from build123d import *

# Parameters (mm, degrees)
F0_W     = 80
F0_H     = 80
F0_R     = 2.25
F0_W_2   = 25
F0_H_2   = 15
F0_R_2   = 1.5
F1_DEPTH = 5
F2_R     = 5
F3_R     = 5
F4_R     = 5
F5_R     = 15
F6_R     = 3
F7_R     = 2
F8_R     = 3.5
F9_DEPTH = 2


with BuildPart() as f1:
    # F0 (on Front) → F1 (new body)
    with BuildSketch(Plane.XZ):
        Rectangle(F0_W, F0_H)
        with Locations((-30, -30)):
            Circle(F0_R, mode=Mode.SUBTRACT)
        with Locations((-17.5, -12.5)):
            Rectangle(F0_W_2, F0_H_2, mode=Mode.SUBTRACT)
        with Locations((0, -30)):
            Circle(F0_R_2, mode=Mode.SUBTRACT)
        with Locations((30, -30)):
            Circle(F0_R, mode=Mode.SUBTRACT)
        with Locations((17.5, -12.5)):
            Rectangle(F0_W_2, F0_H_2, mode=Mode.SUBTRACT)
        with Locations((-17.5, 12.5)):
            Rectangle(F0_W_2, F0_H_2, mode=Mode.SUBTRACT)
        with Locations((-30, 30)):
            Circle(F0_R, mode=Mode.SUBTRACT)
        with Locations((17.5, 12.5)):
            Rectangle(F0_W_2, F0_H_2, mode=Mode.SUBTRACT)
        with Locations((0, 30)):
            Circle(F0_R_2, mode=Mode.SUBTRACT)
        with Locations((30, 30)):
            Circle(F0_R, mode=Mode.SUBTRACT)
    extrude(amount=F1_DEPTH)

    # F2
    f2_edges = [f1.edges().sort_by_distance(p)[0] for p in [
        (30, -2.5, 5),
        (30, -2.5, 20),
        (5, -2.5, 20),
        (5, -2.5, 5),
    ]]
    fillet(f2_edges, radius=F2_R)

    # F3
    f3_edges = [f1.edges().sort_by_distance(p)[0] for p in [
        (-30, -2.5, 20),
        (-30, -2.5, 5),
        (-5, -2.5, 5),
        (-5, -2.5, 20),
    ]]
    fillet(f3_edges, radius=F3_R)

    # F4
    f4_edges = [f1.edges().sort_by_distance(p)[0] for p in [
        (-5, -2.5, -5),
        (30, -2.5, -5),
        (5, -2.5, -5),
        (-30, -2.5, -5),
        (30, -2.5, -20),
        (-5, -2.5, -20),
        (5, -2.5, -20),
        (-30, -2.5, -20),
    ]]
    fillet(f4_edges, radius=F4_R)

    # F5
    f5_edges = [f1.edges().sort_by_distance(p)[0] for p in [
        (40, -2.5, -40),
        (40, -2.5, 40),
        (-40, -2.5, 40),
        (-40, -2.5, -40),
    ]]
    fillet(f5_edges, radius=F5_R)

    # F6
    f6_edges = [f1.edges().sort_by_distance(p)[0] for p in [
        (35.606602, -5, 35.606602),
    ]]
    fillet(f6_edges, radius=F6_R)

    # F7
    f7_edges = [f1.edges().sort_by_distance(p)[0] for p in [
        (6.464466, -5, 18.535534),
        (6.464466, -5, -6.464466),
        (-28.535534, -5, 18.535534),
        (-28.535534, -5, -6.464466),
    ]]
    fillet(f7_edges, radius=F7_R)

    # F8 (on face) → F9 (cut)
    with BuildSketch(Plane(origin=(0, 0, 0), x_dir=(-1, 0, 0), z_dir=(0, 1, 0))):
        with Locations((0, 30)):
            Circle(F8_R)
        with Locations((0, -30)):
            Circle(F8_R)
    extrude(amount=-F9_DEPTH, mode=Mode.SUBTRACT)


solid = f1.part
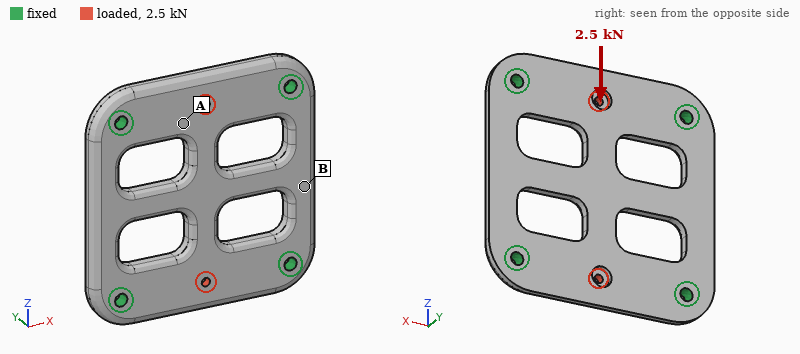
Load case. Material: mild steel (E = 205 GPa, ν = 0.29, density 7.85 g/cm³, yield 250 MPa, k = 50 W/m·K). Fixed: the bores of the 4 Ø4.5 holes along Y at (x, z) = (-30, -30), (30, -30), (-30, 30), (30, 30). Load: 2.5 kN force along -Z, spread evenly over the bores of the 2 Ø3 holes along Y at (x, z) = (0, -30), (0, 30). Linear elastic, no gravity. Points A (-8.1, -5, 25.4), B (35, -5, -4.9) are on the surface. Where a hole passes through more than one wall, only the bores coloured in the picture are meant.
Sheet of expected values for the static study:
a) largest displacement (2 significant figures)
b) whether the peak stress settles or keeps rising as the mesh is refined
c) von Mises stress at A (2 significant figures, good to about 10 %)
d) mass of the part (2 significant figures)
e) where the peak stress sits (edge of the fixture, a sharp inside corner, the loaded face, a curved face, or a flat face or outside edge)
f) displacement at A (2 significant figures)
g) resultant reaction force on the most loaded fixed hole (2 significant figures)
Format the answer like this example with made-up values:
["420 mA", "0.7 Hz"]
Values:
["6.1 µm", "keeps rising", "12 MPa", "180 g", "a sharp inside corner", "4.5 µm", "630 N"]
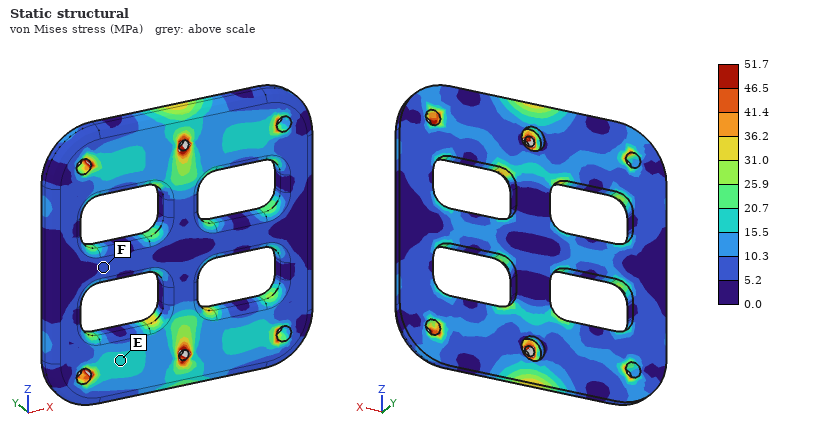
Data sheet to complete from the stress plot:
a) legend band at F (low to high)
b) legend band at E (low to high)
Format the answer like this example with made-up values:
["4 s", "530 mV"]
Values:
["5.2 to 10.3 MPa", "15.5 to 20.7 MPa"]
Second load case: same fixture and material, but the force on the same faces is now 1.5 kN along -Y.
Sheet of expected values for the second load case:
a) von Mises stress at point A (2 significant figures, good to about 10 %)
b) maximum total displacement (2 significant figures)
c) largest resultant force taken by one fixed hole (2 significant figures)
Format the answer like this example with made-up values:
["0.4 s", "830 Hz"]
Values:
["30 MPa", "23 µm", "380 N"]
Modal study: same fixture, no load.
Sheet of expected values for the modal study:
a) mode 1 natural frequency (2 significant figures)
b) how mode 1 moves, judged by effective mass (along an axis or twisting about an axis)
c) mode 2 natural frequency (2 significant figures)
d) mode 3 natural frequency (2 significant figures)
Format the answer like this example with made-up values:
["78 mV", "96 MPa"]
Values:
["4700 Hz", "along Y", "7000 Hz", "7100 Hz"]
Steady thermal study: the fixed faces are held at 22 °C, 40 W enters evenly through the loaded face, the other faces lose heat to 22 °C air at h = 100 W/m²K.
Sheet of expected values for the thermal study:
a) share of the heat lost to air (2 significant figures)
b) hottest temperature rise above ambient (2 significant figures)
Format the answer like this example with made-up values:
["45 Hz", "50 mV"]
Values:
["41 %", "64 K"]
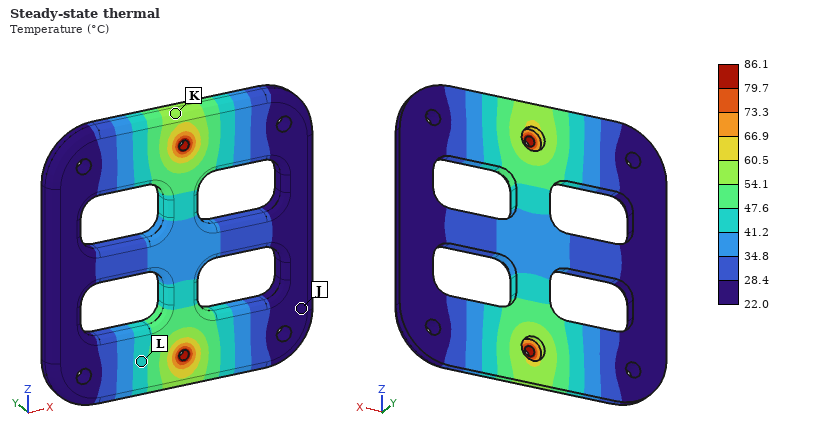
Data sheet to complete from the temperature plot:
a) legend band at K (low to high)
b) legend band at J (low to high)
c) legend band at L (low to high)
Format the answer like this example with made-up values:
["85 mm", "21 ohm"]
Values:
["54.1 to 60.5 °C", "22.0 to 28.4 °C", "41.2 to 47.6 °C"]
